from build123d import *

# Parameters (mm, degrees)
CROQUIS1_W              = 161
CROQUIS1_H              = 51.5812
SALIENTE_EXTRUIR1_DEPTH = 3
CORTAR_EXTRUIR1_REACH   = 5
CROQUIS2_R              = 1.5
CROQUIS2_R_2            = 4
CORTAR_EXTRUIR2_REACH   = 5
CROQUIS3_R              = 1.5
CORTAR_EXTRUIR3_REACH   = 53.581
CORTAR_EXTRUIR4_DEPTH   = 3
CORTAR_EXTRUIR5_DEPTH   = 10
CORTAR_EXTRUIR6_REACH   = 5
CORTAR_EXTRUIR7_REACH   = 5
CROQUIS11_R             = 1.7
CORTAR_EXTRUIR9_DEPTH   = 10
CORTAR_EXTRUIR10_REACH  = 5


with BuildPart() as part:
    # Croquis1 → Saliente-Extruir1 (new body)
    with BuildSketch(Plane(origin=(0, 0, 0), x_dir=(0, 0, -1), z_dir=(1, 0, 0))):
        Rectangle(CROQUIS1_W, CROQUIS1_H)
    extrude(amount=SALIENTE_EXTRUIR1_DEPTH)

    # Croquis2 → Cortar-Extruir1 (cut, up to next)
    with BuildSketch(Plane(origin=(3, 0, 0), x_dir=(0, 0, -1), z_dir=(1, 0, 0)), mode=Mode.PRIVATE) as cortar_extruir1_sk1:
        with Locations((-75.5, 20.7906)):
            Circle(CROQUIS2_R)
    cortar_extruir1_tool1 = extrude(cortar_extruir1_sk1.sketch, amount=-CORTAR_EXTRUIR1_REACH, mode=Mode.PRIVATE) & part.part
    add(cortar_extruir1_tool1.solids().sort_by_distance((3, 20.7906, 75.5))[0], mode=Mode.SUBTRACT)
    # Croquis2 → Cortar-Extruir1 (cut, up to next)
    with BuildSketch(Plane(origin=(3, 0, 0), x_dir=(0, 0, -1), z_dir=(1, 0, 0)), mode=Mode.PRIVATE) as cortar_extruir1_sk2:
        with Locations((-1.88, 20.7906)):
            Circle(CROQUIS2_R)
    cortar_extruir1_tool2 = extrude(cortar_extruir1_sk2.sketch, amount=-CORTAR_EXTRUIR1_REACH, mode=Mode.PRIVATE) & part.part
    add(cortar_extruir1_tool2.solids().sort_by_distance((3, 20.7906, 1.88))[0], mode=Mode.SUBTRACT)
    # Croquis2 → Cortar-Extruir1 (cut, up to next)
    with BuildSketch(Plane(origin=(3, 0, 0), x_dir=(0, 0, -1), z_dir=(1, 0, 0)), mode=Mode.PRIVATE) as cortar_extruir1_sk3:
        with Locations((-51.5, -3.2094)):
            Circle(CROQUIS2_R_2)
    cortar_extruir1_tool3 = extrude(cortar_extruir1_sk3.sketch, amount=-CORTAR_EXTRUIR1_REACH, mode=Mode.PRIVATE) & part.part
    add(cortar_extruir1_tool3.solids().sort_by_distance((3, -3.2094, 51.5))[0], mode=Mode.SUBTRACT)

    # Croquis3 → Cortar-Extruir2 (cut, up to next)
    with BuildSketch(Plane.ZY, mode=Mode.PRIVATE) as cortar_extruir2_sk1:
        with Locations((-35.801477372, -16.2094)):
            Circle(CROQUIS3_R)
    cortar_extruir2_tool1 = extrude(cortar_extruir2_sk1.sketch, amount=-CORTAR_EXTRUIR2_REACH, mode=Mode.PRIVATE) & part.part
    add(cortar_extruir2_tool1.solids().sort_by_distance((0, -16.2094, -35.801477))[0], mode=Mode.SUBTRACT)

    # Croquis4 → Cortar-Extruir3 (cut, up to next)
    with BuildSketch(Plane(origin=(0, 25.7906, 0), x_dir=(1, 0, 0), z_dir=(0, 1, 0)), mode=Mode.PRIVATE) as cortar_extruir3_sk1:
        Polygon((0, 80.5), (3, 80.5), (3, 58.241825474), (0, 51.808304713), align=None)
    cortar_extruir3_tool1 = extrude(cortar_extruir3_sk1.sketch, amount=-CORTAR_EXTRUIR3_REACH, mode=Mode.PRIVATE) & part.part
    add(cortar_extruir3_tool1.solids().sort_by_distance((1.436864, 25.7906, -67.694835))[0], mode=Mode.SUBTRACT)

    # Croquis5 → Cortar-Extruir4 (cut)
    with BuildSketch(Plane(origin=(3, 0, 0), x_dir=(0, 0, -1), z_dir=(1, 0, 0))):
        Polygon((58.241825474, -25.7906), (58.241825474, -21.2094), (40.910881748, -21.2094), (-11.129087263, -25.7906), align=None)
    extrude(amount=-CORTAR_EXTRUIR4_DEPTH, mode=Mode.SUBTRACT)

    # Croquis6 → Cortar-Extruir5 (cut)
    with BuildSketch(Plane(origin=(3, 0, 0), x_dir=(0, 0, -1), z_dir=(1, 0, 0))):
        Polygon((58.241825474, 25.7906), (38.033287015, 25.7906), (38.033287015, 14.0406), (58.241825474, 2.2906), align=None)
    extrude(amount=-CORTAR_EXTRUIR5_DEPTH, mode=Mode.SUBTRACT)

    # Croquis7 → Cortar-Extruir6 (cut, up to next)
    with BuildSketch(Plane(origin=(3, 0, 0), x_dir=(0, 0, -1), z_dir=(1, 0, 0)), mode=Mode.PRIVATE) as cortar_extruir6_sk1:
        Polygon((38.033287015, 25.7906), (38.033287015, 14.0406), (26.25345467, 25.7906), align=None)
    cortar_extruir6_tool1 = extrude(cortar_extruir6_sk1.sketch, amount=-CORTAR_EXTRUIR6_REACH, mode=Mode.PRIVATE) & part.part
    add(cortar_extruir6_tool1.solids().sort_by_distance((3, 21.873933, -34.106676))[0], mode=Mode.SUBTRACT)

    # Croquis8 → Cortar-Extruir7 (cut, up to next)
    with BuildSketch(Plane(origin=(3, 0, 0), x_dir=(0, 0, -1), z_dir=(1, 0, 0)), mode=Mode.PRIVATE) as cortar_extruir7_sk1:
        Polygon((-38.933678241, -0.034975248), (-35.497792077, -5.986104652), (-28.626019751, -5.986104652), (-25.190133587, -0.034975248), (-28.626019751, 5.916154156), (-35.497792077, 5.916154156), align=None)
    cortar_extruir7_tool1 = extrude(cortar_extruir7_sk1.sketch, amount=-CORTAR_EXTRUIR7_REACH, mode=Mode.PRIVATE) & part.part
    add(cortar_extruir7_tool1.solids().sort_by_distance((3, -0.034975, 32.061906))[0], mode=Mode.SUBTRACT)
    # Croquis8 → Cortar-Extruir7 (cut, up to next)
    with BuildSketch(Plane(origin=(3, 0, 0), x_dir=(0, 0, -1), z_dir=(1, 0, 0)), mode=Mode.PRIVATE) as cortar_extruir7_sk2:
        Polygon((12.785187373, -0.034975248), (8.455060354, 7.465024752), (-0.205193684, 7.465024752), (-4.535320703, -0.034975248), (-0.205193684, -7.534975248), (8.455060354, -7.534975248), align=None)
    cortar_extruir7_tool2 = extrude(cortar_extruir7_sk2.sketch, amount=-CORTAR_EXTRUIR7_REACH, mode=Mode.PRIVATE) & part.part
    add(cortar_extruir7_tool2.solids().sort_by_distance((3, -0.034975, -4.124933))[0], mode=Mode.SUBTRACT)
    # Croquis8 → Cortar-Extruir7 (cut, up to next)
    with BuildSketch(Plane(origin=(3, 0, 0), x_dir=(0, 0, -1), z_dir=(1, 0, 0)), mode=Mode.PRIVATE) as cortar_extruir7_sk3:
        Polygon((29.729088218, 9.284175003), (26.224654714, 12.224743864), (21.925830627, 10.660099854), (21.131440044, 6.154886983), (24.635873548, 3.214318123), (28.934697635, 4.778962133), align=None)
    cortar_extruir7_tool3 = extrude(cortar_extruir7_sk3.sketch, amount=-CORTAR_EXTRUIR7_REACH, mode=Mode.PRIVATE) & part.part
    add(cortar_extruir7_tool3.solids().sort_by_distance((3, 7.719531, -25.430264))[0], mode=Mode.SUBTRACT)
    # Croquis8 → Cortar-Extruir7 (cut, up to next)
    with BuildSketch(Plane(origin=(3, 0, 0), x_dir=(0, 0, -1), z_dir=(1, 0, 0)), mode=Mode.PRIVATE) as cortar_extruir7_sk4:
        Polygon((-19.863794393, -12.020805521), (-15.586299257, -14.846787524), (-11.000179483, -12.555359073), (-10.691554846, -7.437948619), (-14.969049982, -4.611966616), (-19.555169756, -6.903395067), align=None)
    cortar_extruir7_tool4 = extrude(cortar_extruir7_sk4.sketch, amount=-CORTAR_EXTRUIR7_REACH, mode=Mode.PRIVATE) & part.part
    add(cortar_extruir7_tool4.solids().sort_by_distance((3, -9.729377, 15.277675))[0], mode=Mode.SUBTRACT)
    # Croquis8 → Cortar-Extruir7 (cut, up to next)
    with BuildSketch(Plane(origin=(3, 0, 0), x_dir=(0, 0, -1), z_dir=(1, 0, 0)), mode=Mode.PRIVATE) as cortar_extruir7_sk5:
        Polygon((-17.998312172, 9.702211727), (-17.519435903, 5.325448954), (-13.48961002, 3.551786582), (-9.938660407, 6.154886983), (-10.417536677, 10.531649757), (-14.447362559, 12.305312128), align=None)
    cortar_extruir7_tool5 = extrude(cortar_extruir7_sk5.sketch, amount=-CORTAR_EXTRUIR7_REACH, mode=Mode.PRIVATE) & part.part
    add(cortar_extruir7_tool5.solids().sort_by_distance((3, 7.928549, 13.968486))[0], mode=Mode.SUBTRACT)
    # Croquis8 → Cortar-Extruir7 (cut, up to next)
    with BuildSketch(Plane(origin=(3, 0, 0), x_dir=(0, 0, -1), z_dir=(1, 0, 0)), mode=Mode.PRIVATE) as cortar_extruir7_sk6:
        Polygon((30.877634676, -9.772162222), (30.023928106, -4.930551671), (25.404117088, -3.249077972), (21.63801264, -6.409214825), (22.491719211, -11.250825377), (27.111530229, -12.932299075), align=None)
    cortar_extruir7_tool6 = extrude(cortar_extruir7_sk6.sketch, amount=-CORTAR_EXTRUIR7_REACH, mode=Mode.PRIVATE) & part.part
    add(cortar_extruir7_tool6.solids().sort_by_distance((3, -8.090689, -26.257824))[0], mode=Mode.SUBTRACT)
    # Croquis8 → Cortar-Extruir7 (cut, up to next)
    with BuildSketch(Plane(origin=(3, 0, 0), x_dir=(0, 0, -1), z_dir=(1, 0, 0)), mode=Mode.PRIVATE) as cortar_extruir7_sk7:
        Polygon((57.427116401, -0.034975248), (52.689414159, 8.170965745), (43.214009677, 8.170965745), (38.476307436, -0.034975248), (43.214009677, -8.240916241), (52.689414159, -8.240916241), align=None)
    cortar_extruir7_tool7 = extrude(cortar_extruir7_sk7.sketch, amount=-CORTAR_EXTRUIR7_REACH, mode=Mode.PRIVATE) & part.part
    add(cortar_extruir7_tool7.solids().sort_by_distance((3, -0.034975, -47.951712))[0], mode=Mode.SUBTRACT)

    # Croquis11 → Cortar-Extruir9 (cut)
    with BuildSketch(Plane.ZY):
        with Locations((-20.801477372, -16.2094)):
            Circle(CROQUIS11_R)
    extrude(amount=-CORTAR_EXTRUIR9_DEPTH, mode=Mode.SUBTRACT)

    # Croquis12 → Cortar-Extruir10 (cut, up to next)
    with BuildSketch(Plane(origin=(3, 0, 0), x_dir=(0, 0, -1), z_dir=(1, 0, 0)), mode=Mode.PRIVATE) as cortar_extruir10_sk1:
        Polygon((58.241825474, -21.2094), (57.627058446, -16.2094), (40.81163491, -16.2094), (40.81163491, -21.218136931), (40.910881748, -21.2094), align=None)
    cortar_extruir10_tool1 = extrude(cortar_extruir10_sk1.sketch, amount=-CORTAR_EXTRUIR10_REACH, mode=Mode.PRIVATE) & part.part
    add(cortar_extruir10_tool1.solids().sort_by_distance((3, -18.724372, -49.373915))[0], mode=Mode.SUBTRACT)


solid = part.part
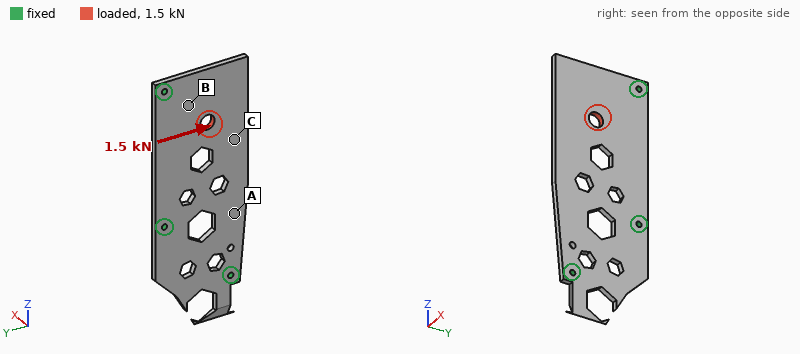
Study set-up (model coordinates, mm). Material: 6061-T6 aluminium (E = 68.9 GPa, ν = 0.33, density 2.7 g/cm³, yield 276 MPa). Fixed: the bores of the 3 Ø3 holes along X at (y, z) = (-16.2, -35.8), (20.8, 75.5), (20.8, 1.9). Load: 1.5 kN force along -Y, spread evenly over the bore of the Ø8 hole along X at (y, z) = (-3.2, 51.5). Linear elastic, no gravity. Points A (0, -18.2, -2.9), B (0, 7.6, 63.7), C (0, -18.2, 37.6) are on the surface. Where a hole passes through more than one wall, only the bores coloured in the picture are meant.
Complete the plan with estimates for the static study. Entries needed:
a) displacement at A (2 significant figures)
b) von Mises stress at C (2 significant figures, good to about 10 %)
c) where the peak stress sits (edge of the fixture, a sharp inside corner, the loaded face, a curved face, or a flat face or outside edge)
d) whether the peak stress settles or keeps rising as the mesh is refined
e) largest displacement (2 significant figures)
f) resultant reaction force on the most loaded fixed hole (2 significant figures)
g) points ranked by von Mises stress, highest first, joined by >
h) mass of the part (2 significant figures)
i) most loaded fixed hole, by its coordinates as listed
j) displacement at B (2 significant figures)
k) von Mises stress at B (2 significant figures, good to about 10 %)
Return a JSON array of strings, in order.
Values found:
["3.2 µm", "10 MPa", "edge of the fixture", "keeps rising", "16 µm", "1.1 kN", "B > C > A", "45 g", "(20.8, 75.5)", "9.4 µm", "17 MPa"]
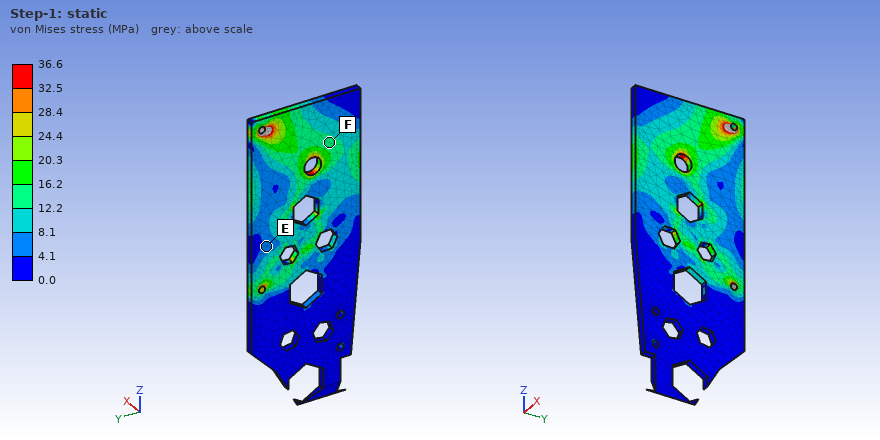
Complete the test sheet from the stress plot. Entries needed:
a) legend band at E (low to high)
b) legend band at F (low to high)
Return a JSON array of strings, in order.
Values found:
["4.1 to 8.1 MPa", "12.2 to 16.2 MPa"]
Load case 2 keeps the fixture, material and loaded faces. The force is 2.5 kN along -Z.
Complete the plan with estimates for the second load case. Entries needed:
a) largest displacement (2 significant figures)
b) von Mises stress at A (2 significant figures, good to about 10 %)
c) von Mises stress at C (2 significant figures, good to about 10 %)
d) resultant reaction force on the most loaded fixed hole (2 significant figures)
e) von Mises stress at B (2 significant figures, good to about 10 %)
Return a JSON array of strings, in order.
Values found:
["22 µm", "12 MPa", "14 MPa", "1.1 kN", "21 MPa"]
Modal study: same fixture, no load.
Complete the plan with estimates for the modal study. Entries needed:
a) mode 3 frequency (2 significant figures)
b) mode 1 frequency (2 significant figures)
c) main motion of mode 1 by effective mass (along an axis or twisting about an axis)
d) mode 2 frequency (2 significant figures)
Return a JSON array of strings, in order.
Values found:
["2900 Hz", "890 Hz", "along X", "2000 Hz"]
